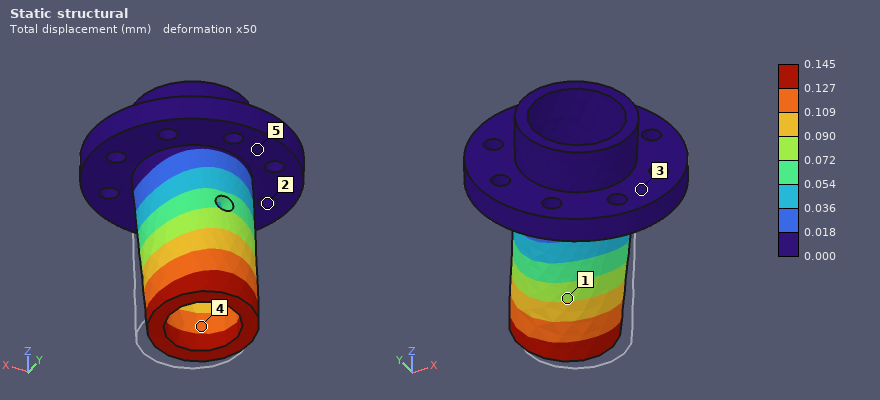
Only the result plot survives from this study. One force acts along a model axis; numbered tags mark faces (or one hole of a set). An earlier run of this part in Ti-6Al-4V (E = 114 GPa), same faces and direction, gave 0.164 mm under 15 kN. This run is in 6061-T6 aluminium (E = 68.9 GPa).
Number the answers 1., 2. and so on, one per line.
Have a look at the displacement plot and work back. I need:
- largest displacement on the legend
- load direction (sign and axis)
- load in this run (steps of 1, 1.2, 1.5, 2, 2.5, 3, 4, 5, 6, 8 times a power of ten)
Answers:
1. 0.145 mm
2. +Y
3. 8 kN
